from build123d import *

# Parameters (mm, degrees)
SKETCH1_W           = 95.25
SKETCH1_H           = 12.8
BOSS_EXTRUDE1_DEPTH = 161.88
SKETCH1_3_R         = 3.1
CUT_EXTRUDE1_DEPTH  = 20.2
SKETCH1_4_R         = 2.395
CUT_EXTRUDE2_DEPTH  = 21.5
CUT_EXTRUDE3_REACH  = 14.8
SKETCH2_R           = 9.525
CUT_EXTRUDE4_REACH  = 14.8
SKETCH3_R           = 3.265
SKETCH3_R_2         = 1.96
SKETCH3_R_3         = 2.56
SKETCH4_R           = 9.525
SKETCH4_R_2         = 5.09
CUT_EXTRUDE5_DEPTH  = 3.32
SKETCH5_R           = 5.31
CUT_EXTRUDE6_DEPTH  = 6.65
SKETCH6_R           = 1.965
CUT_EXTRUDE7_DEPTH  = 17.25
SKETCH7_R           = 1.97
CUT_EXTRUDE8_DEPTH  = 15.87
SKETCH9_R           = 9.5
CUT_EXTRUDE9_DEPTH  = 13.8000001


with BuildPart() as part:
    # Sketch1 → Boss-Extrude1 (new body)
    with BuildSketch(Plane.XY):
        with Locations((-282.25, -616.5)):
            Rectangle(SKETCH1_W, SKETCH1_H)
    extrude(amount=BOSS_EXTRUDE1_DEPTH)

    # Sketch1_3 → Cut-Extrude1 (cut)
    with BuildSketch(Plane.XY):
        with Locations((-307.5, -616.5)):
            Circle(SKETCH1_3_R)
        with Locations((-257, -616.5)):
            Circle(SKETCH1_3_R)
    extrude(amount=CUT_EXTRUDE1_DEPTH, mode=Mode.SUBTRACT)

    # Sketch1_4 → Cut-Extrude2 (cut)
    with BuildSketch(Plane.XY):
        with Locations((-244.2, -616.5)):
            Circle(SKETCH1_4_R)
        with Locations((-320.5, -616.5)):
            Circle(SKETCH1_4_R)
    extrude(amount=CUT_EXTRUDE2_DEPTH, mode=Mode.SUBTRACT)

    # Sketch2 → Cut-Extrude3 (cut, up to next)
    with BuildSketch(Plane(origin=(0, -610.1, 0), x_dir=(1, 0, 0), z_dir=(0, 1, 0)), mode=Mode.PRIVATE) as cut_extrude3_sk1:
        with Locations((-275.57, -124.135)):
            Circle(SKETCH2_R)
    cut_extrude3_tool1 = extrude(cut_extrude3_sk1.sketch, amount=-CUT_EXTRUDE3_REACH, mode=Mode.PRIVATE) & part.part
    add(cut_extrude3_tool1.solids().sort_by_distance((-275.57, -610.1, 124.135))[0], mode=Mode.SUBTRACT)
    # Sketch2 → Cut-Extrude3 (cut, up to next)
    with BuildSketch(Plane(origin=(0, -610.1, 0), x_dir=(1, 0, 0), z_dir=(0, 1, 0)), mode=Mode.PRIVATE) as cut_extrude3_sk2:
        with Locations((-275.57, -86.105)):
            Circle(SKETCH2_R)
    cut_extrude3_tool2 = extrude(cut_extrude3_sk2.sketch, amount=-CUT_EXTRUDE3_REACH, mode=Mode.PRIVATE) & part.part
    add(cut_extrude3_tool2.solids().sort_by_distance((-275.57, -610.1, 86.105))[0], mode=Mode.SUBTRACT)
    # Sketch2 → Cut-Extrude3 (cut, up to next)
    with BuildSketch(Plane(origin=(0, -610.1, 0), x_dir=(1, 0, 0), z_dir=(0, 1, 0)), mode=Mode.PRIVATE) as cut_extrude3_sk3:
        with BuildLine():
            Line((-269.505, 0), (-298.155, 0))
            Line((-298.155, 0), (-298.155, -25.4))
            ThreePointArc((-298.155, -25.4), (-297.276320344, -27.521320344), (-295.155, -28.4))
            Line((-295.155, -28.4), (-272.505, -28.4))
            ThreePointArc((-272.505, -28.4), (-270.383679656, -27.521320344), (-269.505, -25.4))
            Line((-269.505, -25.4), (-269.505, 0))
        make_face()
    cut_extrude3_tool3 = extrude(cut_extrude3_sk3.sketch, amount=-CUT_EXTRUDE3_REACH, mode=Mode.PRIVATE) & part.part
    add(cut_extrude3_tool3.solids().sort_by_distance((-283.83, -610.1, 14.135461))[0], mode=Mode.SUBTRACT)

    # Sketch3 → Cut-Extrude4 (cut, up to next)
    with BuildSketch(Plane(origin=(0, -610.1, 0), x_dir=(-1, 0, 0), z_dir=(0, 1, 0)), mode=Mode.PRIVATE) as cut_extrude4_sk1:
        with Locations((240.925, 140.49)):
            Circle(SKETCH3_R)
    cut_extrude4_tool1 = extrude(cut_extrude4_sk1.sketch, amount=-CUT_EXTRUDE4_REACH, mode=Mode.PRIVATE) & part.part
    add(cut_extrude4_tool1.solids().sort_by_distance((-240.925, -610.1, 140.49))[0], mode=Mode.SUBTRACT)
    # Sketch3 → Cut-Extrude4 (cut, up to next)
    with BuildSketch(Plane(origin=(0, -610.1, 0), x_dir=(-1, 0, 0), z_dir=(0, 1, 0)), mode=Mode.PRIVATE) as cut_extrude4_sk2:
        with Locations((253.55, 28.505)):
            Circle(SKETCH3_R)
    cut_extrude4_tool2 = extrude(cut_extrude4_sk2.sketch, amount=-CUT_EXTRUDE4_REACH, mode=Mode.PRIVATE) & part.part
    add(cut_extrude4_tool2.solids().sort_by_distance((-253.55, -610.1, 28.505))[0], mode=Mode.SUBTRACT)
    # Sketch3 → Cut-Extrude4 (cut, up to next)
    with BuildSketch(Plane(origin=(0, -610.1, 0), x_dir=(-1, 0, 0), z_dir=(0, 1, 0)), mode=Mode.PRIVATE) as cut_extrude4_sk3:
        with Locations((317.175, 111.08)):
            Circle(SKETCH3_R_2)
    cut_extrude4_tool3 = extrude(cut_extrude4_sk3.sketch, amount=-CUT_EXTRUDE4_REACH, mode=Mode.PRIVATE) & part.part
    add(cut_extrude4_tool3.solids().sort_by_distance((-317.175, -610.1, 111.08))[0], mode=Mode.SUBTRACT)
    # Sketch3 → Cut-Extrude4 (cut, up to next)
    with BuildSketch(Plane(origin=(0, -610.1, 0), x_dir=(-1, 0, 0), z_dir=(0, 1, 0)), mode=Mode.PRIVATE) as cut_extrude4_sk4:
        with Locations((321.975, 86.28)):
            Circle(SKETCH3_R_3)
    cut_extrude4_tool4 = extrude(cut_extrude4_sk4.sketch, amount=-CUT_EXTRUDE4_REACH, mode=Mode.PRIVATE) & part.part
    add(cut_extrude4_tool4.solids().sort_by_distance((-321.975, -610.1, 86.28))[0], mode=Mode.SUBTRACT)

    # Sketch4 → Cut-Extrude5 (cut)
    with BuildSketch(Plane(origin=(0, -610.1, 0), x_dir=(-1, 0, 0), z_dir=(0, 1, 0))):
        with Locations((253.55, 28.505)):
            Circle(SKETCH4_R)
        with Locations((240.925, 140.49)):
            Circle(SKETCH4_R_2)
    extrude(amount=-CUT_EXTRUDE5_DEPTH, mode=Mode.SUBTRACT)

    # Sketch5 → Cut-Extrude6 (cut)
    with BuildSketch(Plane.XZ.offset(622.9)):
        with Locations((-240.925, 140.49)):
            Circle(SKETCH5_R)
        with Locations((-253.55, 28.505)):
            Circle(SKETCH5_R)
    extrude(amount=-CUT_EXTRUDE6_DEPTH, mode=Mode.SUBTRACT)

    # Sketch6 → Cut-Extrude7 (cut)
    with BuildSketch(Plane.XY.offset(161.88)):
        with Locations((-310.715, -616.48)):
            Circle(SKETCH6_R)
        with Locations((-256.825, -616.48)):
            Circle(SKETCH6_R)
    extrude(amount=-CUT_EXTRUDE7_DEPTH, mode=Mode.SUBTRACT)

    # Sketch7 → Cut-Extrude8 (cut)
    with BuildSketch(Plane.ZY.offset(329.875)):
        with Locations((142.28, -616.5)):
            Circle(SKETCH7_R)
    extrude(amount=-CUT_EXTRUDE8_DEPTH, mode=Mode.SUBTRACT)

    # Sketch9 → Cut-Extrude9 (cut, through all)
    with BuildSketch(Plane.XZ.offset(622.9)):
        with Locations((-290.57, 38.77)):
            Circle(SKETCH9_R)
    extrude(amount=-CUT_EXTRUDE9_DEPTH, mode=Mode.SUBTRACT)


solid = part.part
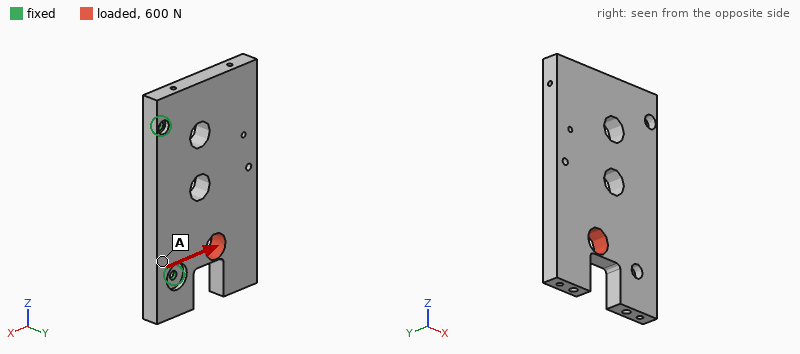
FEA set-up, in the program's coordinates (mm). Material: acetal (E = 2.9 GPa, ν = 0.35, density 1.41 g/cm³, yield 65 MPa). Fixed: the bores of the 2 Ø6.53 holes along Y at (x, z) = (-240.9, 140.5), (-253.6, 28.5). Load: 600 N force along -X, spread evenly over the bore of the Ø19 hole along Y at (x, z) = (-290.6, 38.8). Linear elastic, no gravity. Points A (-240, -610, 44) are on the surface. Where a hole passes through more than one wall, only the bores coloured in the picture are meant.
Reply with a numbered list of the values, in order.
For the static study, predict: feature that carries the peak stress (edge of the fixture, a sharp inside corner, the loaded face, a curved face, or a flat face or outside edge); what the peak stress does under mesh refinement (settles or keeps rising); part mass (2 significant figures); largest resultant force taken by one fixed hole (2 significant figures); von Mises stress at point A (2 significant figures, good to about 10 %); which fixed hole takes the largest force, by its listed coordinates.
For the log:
1. edge of the fixture
2. keeps rising
3. 240 g
4. 540 N
5. 0.94 MPa
6. (-253.6, 28.5)
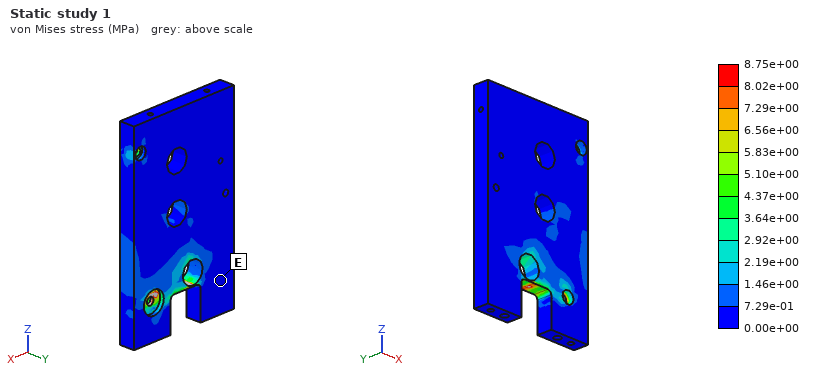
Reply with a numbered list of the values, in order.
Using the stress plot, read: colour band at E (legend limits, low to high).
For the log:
1. 0.00e+00 to 7.29e-01 MPa
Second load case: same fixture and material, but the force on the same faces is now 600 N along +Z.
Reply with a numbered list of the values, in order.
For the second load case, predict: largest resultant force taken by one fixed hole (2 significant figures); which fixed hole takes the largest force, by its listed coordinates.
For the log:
1. 430 N
2. (-253.6, 28.5)
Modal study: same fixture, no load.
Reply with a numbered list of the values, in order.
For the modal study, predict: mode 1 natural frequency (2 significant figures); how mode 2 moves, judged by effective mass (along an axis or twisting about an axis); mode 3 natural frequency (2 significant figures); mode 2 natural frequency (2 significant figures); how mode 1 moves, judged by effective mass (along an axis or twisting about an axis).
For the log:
1. 130 Hz
2. twisting about X
3. 740 Hz
4. 400 Hz
5. along Y
